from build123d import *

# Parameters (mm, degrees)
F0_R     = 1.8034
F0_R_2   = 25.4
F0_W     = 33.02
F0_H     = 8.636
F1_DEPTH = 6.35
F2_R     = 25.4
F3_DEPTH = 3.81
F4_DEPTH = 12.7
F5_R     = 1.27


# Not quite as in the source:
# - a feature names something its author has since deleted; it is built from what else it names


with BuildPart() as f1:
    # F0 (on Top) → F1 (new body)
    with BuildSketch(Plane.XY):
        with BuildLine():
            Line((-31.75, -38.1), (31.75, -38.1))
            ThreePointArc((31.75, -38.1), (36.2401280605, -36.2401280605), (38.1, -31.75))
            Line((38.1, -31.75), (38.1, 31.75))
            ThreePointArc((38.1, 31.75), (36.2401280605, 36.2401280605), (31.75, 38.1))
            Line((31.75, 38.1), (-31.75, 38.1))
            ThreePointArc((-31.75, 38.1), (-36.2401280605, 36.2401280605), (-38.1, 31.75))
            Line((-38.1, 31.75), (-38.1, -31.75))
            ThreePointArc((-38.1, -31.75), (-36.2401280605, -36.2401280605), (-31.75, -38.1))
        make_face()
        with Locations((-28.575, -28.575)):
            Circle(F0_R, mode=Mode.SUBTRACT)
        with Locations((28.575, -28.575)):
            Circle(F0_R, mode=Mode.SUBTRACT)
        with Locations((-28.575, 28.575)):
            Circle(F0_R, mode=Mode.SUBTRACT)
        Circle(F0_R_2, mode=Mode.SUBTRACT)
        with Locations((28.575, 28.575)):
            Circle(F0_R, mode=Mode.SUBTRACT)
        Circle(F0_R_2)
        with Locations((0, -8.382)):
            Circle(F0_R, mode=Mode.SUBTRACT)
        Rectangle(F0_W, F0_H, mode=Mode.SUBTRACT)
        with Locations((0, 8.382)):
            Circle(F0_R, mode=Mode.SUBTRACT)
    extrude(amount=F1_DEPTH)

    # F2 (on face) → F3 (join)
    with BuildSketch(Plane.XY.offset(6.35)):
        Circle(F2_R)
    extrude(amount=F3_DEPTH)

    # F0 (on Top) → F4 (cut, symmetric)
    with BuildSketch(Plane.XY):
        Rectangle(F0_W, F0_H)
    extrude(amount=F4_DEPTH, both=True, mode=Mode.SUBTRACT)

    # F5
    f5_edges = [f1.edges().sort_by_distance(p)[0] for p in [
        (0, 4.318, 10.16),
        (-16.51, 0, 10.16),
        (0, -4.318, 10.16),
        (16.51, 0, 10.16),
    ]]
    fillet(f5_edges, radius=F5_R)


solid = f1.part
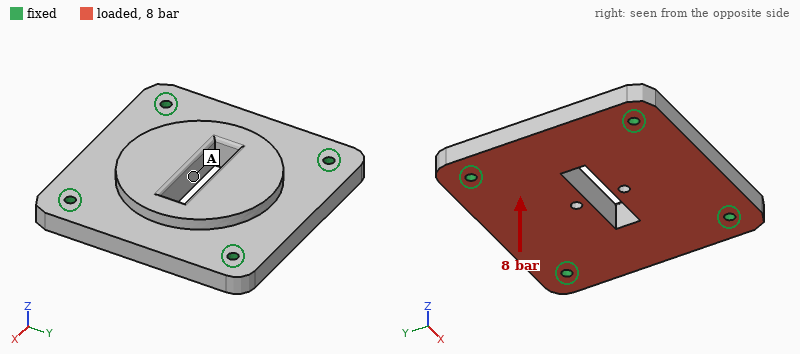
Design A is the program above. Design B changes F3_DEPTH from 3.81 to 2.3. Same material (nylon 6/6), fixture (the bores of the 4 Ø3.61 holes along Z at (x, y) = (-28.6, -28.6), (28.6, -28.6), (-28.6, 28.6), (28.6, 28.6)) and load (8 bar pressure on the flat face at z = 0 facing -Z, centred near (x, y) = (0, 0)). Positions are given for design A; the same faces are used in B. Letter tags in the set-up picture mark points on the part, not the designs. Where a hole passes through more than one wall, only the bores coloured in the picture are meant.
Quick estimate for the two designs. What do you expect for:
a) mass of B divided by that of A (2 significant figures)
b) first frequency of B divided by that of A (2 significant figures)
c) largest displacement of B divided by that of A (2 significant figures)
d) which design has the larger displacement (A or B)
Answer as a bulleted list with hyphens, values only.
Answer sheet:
- 0.94
- 0.97
- 1.3
- B
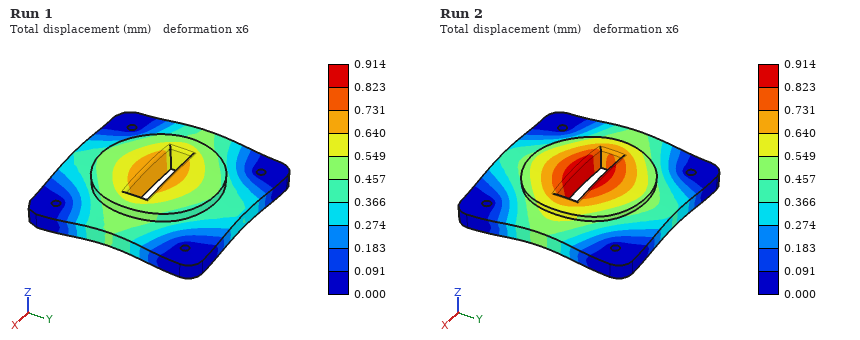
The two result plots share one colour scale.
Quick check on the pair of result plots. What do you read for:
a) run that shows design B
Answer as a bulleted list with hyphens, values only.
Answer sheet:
- Run 2
